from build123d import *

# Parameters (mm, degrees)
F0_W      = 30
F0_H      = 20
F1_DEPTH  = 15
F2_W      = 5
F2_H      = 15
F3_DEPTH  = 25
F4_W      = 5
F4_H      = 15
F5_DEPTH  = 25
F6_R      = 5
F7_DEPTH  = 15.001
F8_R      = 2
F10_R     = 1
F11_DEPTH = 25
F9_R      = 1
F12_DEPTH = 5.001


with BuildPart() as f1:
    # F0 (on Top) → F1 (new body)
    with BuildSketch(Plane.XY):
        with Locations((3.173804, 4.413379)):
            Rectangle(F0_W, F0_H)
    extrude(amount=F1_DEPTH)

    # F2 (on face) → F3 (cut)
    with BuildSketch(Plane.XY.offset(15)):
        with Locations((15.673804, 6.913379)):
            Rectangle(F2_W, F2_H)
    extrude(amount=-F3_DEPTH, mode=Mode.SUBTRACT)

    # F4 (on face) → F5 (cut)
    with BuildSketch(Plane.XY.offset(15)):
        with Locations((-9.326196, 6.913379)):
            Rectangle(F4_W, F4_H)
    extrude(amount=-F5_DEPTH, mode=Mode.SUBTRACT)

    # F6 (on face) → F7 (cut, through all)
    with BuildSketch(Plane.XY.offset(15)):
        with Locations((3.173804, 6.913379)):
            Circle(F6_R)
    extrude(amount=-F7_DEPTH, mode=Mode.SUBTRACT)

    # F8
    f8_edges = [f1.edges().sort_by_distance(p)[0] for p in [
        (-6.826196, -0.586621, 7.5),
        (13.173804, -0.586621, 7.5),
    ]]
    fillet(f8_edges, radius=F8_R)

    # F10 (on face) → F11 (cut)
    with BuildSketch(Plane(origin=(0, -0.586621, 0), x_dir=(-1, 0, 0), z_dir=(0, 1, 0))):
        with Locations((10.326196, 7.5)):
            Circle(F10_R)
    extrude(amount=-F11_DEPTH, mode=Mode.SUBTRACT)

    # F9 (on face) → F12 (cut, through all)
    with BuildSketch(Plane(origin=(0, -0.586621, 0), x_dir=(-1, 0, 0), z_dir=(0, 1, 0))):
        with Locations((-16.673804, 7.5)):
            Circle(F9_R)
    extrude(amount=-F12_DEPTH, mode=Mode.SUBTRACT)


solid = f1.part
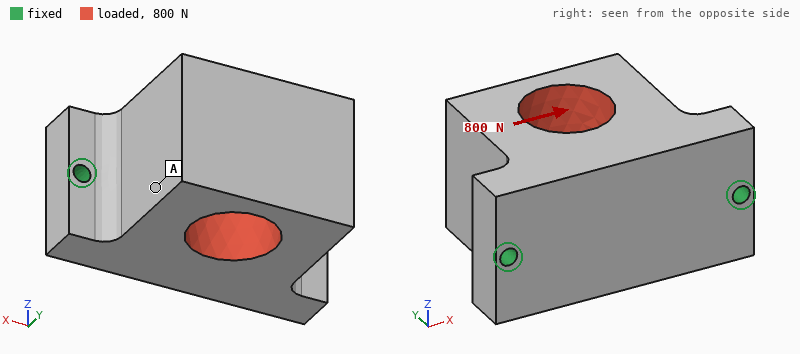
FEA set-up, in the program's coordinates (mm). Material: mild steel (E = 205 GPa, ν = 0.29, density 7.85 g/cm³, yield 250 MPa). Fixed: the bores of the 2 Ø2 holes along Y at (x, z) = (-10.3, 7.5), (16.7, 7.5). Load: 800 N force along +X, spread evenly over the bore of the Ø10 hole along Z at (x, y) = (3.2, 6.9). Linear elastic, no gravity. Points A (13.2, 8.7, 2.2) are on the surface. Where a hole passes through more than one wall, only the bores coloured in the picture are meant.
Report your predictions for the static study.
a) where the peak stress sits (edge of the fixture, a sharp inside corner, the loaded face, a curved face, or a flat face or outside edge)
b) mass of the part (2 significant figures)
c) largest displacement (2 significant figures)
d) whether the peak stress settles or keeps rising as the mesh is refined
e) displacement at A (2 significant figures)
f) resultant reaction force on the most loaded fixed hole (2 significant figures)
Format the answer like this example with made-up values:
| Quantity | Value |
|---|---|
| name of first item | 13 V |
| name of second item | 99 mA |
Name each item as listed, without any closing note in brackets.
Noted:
| Quantity | Value |
|---|---|
| where the peak stress sits | edge of the fixture |
| mass of the part | 44 g |
| largest displacement | 2.5 µm |
| whether the peak stress settles or keeps rising as the mesh is refined | keeps rising |
| displacement at A | 1.8 µm |
| resultant reaction force on the most loaded fixed hole | 510 N |
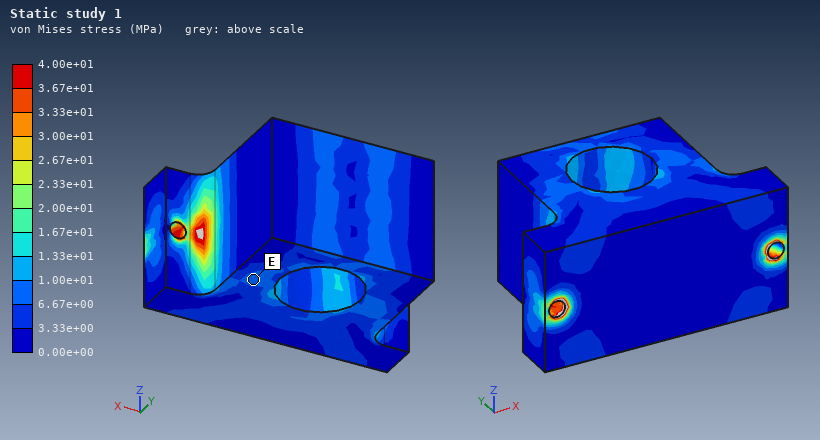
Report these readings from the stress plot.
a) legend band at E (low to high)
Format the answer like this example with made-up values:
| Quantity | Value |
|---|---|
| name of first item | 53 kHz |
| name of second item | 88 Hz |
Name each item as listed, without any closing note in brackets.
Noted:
| Quantity | Value |
|---|---|
| legend band at E | 6.67e+00 to 1.00e+01 MPa |
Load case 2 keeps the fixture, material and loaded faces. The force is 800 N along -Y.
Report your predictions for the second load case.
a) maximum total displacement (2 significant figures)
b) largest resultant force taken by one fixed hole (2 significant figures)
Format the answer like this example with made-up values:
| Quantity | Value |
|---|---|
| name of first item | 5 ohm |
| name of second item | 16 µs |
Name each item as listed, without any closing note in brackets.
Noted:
| Quantity | Value |
|---|---|
| maximum total displacement | 1.3 µm |
| largest resultant force taken by one fixed hole | 430 N |
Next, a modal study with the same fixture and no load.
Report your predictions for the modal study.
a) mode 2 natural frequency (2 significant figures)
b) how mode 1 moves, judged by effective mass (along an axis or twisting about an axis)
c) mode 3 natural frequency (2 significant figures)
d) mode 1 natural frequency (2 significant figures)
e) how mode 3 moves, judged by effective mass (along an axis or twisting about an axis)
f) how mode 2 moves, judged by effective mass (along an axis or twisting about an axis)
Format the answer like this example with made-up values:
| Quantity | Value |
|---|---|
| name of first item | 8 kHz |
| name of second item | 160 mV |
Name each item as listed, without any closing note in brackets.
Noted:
| Quantity | Value |
|---|---|
| mode 2 natural frequency | 20 kHz |
| how mode 1 moves, judged by effective mass | along Z |
| mode 3 natural frequency | 21 kHz |
| mode 1 natural frequency | 8100 Hz |
| how mode 3 moves, judged by effective mass | along Y |
| how mode 2 moves, judged by effective mass | along X |
